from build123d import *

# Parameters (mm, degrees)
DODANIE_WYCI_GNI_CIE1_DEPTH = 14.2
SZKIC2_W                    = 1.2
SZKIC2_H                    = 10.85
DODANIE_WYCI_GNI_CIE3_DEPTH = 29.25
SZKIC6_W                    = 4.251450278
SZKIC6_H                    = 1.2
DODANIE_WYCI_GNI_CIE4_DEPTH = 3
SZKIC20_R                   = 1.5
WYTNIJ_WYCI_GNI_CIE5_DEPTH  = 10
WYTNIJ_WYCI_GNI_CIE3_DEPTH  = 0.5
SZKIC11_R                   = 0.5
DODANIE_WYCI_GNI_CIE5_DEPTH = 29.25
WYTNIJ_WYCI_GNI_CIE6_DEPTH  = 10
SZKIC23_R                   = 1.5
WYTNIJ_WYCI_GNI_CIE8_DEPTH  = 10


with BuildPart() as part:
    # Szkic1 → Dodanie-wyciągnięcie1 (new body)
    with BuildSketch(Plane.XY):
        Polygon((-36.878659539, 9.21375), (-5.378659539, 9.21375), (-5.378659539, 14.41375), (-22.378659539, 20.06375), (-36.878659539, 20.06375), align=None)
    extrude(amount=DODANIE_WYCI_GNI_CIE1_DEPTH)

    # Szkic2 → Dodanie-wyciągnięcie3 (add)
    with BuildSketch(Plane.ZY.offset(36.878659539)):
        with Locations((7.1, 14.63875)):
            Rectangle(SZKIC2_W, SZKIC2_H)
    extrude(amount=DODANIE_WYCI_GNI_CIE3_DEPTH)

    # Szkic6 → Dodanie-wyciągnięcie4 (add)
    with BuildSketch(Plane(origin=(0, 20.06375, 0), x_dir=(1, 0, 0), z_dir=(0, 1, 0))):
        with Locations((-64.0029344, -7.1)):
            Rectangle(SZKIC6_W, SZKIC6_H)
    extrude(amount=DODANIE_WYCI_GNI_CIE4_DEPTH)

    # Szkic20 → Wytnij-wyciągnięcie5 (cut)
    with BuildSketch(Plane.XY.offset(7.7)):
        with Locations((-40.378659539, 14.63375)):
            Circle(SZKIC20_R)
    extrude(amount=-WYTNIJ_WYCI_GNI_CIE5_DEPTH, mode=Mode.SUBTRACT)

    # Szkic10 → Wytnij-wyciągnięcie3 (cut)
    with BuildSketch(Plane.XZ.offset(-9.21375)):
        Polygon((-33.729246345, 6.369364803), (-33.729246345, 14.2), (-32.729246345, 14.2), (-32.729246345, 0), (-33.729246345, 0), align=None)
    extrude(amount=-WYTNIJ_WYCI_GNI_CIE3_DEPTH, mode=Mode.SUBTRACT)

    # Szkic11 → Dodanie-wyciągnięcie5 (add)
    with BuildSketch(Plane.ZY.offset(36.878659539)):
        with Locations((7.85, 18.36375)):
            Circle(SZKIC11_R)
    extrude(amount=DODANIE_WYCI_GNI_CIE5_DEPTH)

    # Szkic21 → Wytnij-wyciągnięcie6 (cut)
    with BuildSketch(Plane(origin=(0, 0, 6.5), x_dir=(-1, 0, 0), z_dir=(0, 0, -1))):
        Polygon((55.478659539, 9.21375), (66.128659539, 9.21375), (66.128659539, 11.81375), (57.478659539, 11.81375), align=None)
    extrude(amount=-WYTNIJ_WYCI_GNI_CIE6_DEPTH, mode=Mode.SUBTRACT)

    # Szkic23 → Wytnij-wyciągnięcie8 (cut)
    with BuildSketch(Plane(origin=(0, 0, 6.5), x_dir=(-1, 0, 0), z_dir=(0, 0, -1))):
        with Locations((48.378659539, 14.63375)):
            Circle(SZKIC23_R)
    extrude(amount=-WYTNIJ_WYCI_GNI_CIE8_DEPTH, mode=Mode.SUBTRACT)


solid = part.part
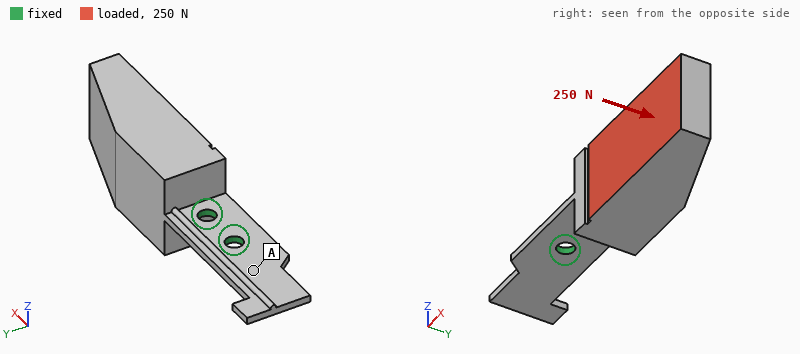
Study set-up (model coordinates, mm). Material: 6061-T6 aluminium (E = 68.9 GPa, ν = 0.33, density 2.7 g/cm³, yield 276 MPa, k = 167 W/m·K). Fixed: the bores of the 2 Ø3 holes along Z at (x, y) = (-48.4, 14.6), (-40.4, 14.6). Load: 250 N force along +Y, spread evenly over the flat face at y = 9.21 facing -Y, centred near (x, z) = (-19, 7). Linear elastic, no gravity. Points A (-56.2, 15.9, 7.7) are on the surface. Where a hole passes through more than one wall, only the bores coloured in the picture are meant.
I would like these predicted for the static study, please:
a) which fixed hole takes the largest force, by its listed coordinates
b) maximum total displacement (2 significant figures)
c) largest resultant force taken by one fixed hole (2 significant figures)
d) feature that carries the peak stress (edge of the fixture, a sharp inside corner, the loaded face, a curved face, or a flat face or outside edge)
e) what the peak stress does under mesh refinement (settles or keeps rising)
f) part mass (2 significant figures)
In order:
(-40.4, 14.6)
0.18 mm
590 N
edge of the fixture
keeps rising
12 g
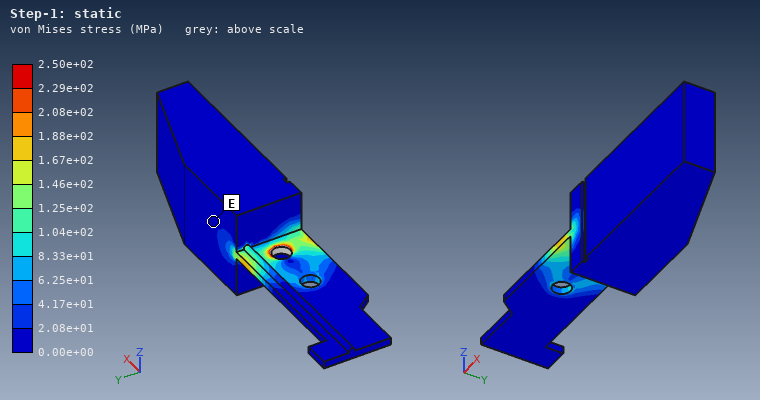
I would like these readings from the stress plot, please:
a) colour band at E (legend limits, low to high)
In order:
0.00e+00 to 2.08e+01 MPa
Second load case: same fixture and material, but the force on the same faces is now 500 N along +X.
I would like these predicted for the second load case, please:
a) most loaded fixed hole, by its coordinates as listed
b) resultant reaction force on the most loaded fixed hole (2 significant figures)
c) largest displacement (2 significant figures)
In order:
(-40.4, 14.6)
470 N
100 µm
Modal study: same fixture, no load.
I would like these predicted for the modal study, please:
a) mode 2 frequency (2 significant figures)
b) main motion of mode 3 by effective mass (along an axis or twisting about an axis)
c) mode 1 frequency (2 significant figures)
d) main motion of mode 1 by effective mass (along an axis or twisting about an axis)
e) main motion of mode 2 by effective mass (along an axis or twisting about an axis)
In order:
2600 Hz
twisting about X
540 Hz
along Z
along Y
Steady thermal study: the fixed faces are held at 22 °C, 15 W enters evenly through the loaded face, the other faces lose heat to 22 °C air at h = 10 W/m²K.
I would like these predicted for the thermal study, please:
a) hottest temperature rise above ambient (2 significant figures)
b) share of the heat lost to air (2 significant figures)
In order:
39 K
3.1 %
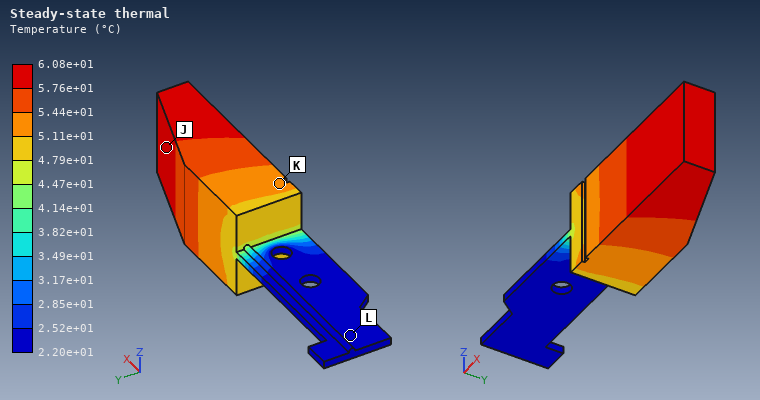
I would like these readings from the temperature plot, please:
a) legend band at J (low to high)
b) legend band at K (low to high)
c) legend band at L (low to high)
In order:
5.76e+01 to 6.08e+01 °C
5.11e+01 to 5.44e+01 °C
2.20e+01 to 2.52e+01 °C
